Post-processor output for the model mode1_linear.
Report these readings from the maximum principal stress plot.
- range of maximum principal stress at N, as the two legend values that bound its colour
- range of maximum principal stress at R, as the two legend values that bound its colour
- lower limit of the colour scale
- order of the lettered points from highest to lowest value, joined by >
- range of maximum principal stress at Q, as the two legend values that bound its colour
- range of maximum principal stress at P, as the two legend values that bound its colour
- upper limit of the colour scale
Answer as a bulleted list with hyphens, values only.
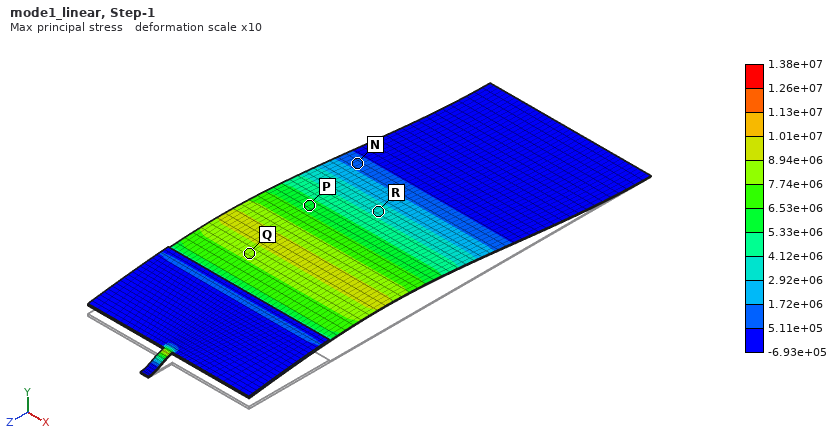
- 5.11e+05 to 1.72e+06
- 2.92e+06 to 4.12e+06
- -6.93e+05
- Q > P > R > N
- 7.74e+06 to 8.94e+06
- 5.33e+06 to 6.53e+06
- 1.38e+07
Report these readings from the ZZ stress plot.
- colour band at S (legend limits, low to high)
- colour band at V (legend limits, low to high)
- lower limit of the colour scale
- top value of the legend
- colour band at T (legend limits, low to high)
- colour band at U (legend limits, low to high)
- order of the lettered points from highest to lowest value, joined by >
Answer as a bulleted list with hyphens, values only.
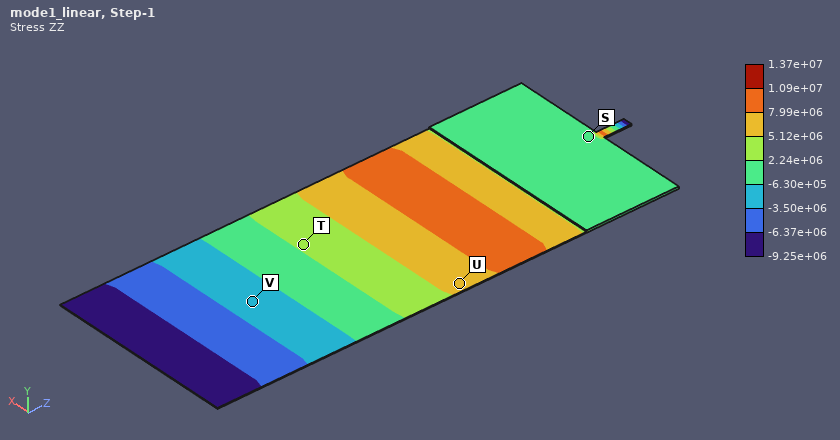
- -6.30e+05 to 2.24e+06
- -3.50e+06 to -6.30e+05
- -9.25e+06
- 1.37e+07
- 2.24e+06 to 5.12e+06
- 5.12e+06 to 7.99e+06
- U > T > S > V
